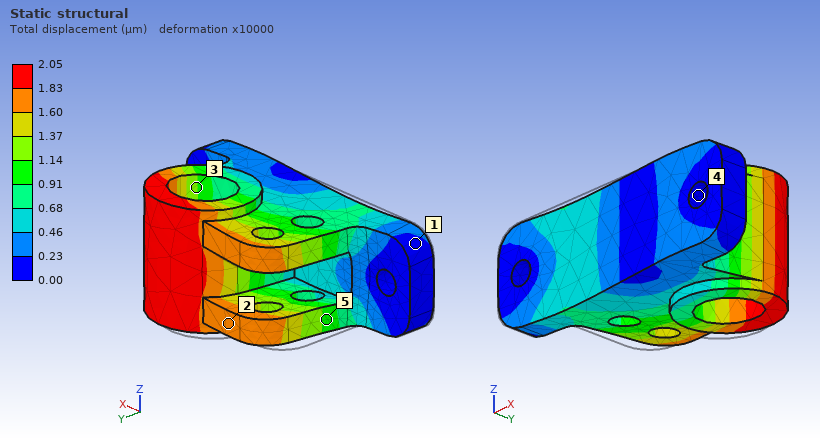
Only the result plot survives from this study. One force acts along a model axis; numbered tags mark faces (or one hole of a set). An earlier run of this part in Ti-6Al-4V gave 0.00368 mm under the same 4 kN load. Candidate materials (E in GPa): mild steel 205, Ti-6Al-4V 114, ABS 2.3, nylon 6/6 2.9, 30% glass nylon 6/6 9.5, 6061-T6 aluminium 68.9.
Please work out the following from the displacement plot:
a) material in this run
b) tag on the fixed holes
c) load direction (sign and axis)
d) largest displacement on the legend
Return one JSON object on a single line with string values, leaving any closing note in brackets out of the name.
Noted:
{"material in this run": "mild steel", "tag on the fixed holes": "4", "load direction": "+X", "largest displacement on the legend": "2.05 µm"}
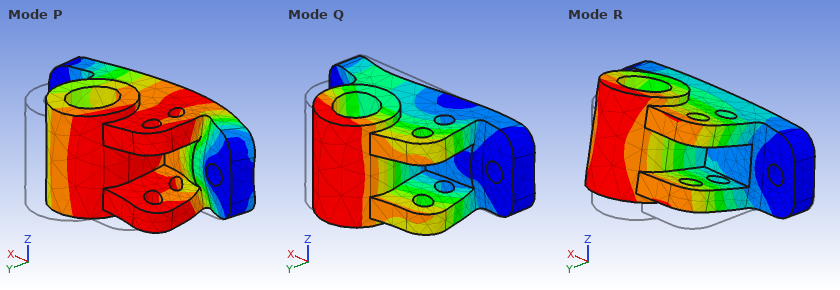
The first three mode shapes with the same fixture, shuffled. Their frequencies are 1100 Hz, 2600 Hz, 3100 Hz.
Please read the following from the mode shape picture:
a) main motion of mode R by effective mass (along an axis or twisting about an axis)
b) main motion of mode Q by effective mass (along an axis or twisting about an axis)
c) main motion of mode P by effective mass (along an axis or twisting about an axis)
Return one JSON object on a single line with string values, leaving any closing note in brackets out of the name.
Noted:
{"main motion of mode R by effective mass": "along Z", "main motion of mode Q by effective mass": "along X", "main motion of mode P by effective mass": "along Y"}
